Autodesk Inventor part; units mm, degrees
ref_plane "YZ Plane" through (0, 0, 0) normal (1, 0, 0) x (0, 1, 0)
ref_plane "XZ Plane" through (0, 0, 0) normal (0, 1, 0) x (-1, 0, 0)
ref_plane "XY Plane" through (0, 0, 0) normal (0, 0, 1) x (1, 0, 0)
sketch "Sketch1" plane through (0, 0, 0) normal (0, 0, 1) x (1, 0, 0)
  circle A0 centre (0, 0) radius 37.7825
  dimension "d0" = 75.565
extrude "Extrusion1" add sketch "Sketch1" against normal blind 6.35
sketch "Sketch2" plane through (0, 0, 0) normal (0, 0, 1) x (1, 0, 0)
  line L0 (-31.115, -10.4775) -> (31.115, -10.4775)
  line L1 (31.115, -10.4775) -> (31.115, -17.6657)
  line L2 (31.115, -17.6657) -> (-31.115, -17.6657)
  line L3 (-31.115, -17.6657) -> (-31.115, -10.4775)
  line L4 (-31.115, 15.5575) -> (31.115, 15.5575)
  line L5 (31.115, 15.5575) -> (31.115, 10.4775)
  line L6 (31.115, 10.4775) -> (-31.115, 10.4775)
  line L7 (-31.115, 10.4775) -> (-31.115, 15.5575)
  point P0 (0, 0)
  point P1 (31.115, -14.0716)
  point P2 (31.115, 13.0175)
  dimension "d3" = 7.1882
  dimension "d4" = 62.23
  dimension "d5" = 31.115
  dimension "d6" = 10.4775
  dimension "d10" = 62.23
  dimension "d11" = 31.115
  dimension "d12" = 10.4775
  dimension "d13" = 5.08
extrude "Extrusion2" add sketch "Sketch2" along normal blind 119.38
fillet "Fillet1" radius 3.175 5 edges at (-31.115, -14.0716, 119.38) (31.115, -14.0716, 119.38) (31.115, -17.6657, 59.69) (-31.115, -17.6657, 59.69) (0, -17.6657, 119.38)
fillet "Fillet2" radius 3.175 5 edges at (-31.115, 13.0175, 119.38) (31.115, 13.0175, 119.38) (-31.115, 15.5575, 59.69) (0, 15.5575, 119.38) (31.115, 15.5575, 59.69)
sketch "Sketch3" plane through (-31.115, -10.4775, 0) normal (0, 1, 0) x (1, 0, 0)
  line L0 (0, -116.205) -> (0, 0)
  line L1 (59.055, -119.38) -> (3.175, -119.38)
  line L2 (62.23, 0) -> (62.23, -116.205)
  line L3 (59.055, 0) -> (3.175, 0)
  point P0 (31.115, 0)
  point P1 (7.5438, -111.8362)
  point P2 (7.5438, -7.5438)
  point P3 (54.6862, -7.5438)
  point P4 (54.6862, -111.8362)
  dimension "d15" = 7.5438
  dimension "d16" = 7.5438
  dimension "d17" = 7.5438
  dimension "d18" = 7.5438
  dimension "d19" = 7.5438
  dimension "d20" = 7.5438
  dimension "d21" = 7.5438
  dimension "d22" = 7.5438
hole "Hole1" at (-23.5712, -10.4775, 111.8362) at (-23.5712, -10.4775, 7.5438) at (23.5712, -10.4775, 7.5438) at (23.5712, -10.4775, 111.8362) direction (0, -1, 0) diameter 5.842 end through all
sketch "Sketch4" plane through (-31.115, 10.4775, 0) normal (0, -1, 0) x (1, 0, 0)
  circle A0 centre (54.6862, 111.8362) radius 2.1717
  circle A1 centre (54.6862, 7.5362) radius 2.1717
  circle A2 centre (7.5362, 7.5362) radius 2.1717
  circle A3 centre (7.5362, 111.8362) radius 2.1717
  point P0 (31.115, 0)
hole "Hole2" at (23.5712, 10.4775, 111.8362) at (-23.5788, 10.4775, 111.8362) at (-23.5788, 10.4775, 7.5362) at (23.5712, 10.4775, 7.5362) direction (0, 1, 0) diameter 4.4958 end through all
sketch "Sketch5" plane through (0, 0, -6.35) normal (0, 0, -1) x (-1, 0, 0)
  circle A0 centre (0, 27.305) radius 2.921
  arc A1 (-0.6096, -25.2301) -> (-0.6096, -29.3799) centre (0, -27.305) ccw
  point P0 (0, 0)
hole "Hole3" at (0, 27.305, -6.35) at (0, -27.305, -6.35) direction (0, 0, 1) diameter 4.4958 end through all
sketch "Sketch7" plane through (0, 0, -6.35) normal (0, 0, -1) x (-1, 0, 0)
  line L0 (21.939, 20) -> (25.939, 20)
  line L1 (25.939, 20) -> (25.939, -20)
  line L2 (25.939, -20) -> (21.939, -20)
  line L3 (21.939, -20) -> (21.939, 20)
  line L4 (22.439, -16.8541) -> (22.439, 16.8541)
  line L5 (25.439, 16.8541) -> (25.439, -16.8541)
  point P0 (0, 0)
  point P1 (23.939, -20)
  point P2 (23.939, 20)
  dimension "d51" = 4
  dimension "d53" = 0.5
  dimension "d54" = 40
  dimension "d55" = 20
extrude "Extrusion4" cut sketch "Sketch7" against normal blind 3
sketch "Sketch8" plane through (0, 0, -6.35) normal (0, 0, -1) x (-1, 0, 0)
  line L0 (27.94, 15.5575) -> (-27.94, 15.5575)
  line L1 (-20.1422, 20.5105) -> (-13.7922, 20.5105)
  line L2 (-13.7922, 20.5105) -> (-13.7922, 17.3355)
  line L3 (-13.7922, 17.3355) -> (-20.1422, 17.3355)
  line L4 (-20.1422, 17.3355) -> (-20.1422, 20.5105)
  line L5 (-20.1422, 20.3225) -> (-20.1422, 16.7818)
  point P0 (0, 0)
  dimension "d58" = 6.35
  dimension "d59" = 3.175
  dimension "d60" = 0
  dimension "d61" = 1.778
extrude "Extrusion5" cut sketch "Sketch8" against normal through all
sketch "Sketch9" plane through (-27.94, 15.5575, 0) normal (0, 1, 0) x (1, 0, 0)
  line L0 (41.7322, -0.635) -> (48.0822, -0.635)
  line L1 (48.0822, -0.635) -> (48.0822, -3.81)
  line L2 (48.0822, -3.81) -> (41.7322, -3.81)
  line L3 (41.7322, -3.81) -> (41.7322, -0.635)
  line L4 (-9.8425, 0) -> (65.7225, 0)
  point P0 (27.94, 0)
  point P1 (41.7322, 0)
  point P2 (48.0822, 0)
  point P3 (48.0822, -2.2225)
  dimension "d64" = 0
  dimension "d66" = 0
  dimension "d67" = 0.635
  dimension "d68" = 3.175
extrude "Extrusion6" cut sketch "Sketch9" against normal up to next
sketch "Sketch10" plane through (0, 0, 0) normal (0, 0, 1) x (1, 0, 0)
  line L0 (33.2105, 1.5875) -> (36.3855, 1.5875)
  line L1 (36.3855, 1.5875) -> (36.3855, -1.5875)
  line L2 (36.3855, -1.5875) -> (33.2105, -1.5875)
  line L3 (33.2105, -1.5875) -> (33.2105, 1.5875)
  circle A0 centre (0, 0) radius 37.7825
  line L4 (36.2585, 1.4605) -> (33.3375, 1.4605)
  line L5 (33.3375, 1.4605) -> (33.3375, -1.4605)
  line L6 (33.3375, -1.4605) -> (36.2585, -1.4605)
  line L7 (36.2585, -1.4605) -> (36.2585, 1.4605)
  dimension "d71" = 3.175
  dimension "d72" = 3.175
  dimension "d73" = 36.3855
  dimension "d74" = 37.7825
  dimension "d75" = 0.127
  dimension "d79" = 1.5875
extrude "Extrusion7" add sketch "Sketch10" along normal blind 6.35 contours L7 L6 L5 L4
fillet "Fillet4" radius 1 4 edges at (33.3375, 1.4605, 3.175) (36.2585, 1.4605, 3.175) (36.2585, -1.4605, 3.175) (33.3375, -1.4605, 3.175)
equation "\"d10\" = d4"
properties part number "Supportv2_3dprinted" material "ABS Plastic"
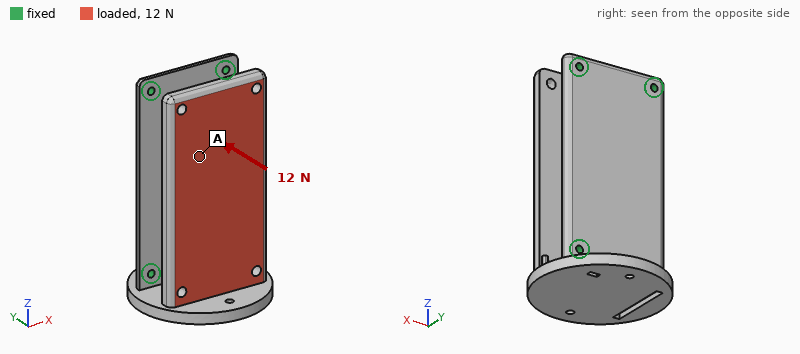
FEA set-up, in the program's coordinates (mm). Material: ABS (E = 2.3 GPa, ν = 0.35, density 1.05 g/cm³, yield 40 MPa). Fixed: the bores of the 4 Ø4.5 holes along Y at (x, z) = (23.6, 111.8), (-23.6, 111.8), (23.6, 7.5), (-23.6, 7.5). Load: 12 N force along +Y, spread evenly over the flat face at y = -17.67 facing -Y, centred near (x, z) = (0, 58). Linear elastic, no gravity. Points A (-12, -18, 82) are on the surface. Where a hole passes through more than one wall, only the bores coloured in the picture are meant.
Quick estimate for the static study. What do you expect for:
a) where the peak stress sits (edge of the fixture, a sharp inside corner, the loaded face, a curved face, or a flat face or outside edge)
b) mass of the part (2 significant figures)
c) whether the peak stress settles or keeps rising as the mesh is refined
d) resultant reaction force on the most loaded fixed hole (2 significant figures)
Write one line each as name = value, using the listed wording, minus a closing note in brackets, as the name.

where the peak stress sits = edge of the fixture
mass of the part = 120 g
whether the peak stress settles or keeps rising as the mesh is refined = keeps rising
resultant reaction force on the most loaded fixed hole = 6.4 N
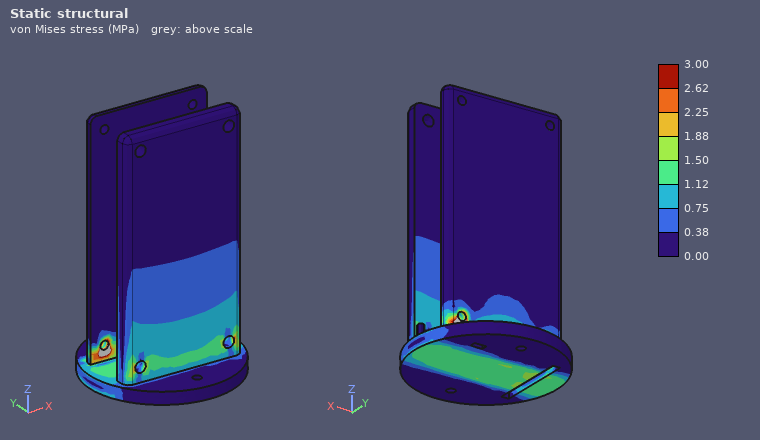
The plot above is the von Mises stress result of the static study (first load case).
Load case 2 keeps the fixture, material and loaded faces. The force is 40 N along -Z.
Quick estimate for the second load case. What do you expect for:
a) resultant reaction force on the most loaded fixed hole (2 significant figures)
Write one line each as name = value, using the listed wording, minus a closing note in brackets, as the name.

resultant reaction force on the most loaded fixed hole = 18 N
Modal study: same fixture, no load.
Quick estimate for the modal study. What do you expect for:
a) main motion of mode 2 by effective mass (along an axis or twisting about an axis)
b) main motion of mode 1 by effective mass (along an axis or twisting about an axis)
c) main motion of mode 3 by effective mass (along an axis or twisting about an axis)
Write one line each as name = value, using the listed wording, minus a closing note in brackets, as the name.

main motion of mode 2 by effective mass = along X
main motion of mode 1 by effective mass = along Y
main motion of mode 3 by effective mass = along Z
